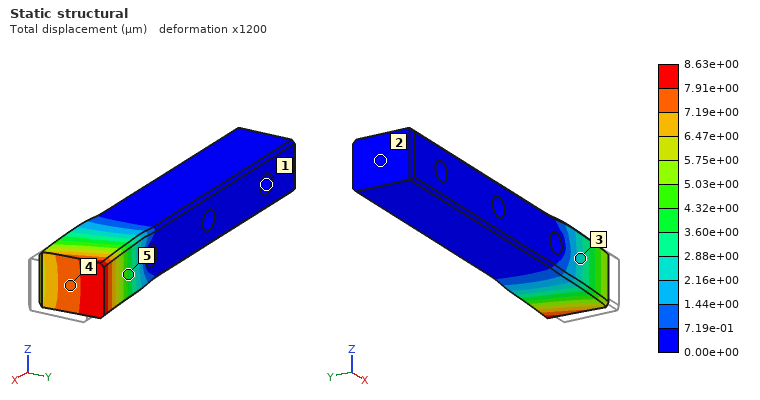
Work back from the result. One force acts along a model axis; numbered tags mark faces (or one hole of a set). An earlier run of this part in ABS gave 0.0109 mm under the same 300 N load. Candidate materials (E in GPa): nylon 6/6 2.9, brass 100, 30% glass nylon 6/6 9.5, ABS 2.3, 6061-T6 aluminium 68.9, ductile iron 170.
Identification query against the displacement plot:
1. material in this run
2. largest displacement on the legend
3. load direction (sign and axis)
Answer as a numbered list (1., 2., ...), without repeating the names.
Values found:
1. nylon 6/6
2. 8.63e+00 µm
3. -X
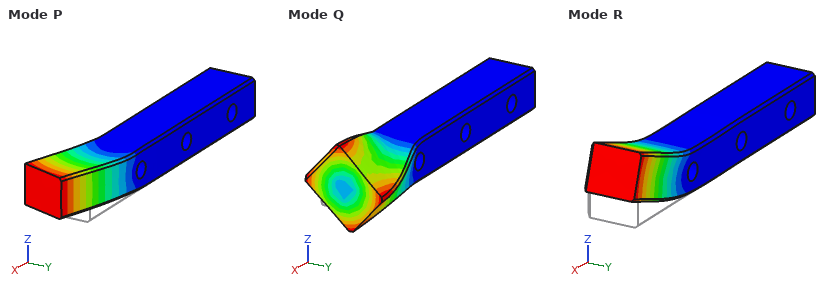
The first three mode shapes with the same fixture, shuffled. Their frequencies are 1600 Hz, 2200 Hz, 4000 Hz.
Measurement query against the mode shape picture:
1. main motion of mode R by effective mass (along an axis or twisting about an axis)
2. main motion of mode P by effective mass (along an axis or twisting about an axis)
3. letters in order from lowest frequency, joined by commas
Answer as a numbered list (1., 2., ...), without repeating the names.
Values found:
1. along Z
2. along Y
3. R, P, Q
